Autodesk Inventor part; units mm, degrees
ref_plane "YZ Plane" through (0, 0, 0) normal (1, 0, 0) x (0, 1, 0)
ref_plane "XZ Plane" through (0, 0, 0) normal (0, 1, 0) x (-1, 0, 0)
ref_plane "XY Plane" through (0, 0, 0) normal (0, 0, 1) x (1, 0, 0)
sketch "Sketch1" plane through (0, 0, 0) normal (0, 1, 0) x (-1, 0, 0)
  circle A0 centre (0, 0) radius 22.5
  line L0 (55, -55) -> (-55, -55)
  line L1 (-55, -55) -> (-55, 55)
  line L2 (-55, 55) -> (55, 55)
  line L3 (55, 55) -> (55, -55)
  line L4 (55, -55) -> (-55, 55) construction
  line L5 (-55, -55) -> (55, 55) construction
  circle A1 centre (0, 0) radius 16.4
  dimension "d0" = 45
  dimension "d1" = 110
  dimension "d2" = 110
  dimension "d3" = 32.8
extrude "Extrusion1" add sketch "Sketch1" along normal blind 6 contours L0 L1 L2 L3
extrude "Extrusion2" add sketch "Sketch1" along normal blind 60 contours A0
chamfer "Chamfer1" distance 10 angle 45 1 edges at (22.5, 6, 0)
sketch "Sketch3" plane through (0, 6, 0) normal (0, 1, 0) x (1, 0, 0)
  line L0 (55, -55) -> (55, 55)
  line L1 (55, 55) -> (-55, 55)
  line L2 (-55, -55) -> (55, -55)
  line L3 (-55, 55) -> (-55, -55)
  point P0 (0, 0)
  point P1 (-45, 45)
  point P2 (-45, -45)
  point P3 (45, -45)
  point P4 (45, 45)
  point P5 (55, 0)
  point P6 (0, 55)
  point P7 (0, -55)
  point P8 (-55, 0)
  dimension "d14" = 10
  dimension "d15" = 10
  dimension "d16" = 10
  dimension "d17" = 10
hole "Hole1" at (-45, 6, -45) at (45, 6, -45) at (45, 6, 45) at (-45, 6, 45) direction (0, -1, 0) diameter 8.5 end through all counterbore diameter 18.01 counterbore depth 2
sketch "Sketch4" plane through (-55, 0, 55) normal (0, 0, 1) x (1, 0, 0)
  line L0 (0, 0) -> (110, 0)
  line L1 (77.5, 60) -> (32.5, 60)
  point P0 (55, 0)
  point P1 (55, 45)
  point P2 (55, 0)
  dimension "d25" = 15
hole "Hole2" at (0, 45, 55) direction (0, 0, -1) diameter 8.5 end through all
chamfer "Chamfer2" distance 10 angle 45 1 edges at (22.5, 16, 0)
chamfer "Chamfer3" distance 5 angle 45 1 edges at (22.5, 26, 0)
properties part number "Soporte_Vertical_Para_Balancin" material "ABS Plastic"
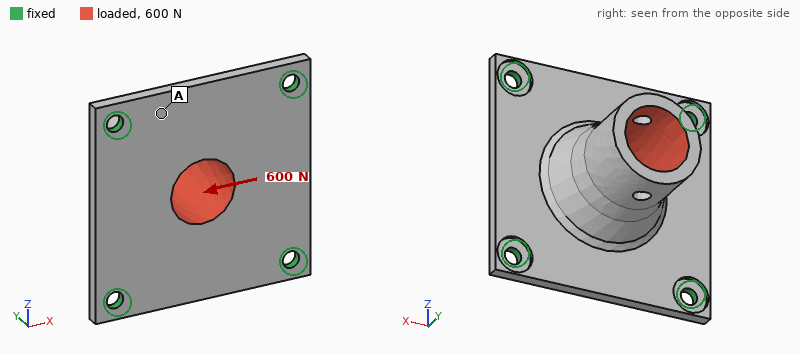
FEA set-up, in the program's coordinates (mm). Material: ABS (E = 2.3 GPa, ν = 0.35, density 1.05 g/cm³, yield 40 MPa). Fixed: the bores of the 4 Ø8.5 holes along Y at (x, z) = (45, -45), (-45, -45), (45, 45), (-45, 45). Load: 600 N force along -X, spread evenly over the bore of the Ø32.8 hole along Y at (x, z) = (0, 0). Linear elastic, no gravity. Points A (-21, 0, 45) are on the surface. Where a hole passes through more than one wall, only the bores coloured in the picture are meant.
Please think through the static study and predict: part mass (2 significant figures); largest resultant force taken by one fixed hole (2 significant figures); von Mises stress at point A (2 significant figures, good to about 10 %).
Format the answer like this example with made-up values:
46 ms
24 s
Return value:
120 g
230 N
1.7 MPa
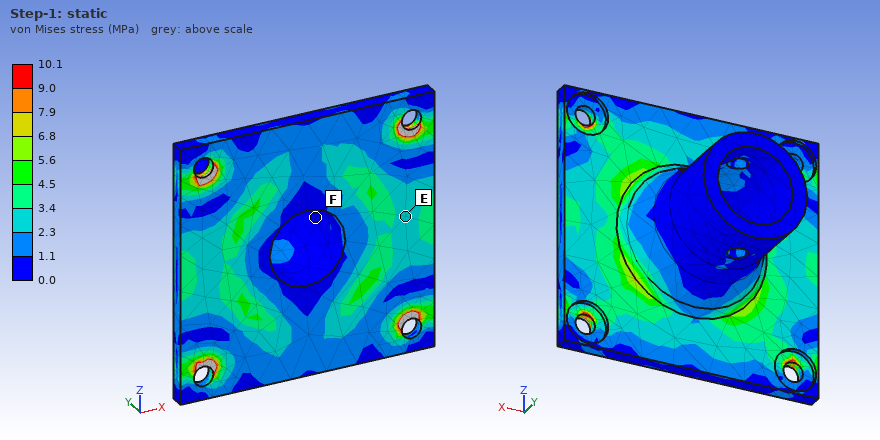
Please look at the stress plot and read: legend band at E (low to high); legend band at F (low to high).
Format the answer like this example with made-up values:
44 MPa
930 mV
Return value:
2.3 to 3.4 MPa
0.0 to 1.1 MPa
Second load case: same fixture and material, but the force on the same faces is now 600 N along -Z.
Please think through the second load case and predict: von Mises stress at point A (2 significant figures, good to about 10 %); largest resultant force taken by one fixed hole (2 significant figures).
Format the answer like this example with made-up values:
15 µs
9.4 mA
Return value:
1.7 MPa
230 N
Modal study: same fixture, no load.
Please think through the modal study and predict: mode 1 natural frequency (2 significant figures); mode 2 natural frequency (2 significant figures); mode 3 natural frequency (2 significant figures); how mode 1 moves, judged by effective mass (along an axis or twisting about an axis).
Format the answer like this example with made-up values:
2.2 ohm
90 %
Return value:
620 Hz
750 Hz
750 Hz
along Y
